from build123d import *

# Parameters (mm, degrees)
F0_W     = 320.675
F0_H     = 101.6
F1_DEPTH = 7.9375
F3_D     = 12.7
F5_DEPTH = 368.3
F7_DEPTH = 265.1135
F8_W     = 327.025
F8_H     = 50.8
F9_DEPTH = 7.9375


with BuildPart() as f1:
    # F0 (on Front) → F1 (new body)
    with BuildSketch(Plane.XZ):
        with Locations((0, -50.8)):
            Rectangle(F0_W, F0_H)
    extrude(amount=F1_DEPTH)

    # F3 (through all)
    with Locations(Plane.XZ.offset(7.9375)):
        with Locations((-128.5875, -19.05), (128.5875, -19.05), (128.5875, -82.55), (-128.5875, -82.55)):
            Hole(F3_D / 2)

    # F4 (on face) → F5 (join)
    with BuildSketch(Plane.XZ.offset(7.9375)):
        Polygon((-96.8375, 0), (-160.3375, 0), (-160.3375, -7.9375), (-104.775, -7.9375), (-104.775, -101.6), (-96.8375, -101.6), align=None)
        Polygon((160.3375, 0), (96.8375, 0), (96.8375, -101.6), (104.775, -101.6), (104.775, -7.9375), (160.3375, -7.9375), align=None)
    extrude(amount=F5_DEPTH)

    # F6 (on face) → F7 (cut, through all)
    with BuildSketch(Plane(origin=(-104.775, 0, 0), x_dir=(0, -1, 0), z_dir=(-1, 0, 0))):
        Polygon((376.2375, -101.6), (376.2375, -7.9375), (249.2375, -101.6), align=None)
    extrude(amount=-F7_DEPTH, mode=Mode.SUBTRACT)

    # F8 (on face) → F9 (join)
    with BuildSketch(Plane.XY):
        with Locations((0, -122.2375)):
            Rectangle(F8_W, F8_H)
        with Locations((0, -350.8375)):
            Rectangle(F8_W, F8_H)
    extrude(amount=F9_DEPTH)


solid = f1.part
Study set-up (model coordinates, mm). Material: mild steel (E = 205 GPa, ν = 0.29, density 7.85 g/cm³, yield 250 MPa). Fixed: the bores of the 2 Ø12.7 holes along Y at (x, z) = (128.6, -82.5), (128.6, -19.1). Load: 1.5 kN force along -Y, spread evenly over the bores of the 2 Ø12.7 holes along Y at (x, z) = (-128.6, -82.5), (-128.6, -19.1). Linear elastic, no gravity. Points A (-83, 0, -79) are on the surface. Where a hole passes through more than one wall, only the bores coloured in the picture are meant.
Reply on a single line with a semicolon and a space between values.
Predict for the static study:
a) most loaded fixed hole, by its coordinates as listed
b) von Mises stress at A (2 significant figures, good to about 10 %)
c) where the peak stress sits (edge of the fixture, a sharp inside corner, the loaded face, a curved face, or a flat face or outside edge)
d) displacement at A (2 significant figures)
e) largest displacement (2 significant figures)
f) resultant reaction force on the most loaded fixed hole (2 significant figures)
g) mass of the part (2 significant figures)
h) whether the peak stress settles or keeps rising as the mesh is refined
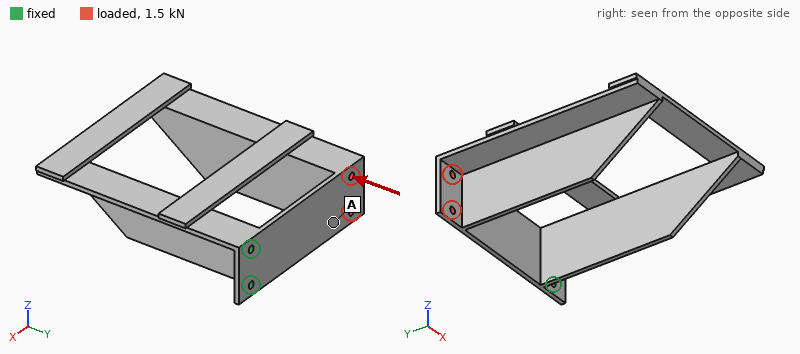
(128.6, -19.1); 16 MPa; edge of the fixture; 0.90 mm; 1.9 mm; 1.1 kN; 11 kg; keeps rising
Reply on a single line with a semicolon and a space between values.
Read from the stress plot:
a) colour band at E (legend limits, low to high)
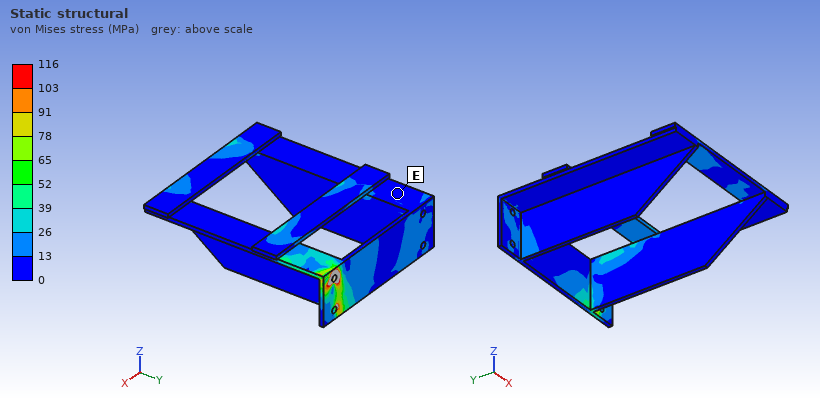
0 to 13 MPa
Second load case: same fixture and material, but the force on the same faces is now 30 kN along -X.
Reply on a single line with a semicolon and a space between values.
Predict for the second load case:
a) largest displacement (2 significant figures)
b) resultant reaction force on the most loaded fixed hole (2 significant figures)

74 µm; 15 kN
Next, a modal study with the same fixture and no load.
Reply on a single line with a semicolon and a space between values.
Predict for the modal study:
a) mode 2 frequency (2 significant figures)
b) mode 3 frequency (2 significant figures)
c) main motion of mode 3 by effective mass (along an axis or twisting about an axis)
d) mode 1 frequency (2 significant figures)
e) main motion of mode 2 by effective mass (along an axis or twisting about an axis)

73 Hz; 240 Hz; along Z; 58 Hz; along Z
